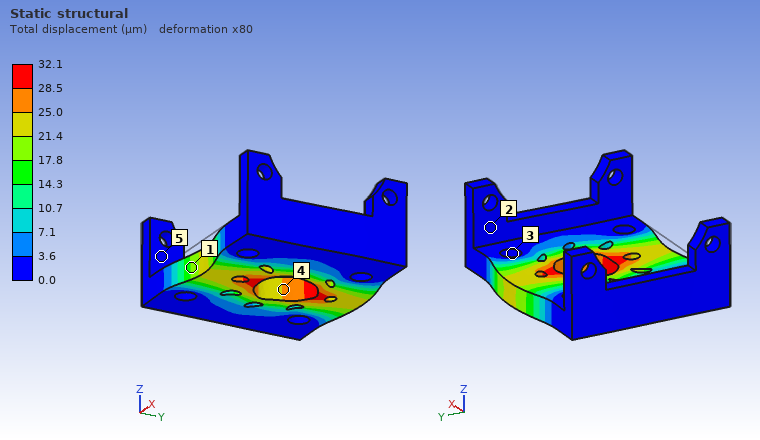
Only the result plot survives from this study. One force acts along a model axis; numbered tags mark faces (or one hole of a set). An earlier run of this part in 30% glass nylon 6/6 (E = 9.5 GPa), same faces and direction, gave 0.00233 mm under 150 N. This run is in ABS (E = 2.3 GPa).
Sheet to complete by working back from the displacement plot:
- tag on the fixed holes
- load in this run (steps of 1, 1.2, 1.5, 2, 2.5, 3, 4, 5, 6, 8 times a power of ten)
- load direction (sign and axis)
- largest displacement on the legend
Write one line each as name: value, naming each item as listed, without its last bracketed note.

tag on the fixed holes: 3
load in this run: 500 N
load direction: +Y
largest displacement on the legend: 32.1 µm
